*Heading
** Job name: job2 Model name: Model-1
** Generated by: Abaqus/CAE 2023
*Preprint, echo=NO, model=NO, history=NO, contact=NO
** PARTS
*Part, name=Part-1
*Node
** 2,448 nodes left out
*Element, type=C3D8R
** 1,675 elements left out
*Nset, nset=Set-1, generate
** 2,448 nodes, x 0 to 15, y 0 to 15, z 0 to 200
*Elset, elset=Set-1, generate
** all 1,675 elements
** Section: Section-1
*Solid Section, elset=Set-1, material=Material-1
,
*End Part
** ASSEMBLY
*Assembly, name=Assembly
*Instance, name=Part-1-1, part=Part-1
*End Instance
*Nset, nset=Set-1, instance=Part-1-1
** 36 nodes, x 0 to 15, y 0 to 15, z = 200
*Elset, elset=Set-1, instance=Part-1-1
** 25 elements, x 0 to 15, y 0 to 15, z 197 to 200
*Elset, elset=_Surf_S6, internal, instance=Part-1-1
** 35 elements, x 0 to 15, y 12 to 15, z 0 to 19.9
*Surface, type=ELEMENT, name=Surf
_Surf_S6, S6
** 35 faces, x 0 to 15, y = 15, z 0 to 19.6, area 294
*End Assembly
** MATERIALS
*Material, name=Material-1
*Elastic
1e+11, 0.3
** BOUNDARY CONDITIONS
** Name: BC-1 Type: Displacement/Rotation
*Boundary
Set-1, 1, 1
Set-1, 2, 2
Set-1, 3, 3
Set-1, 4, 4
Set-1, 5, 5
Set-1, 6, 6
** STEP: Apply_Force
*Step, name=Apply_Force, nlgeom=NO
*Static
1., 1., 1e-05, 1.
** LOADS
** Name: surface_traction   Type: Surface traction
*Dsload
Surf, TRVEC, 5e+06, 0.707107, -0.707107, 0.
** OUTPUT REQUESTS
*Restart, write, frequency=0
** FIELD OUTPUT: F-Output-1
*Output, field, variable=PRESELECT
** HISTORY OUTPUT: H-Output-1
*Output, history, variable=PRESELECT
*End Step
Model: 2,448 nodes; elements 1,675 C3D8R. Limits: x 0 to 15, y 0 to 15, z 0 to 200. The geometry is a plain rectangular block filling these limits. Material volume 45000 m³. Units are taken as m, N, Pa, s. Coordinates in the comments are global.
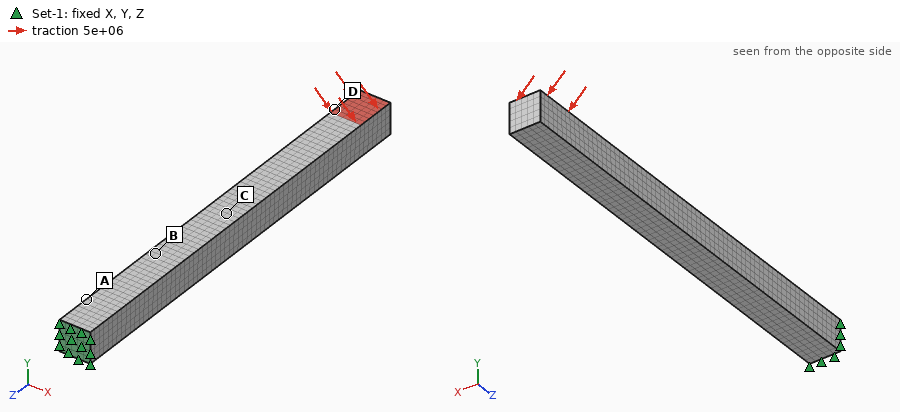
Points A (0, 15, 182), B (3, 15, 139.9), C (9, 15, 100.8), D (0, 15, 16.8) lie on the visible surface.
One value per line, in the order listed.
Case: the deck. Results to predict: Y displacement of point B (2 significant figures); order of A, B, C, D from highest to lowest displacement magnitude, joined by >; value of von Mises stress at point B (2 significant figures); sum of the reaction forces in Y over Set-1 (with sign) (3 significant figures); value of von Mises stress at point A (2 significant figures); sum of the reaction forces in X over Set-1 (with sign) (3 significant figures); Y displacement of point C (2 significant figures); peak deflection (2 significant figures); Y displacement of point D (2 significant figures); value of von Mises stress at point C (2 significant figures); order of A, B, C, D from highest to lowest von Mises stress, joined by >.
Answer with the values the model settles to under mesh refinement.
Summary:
-0.75 m
D > C > B > A
3.9e+08 Pa
1.04e+09 N
6.4e+08 Pa
-1.04e+09 N
-1.9 m
8.7 m
-5.3 m
1.4e+08 Pa
A > B > C > D
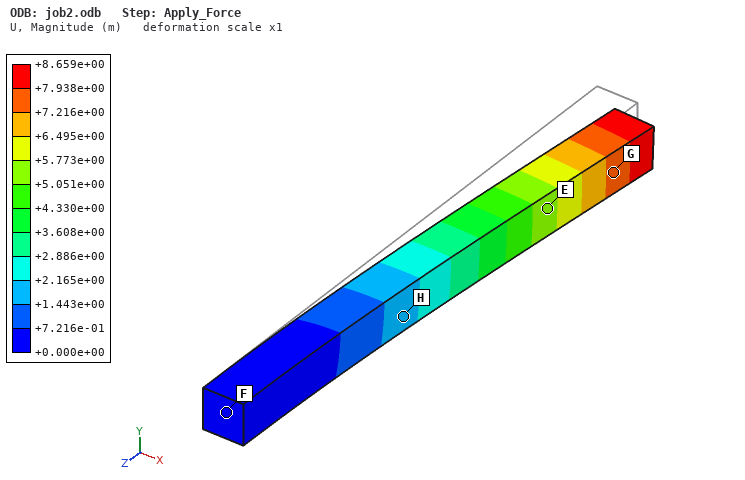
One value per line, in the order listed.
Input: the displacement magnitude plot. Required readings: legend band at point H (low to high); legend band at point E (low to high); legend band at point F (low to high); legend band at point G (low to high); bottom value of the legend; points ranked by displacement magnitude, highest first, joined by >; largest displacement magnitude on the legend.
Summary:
+1.443e+00 to +2.165e+00 m
+5.051e+00 to +5.773e+00 m
+0.000e+00 to +7.216e-01 m
+7.216e+00 to +7.938e+00 m
+0.000e+00 m
G > E > H > F
+8.659e+00 m
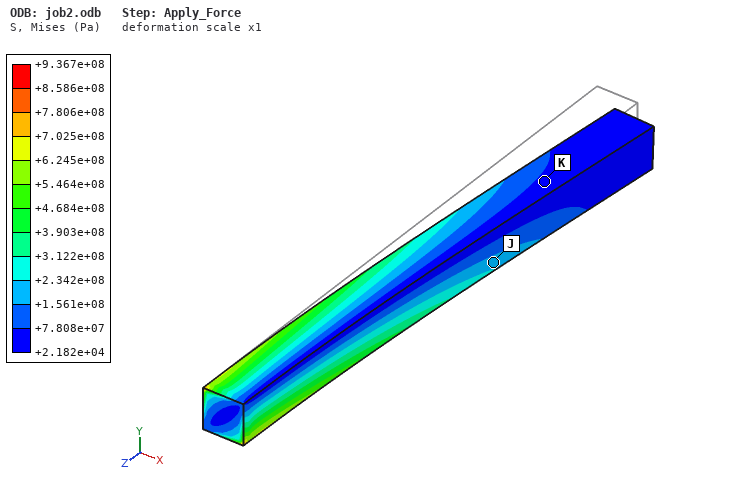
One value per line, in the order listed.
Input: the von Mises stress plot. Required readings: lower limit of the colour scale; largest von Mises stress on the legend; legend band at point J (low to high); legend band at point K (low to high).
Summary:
+2.182e+04 Pa
+9.367e+08 Pa
+1.561e+08 to +2.342e+08 Pa
+2.182e+04 to +7.808e+07 Pa
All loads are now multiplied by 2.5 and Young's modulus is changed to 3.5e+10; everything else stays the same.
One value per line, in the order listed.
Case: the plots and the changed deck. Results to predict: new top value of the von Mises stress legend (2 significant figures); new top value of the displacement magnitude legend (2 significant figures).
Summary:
2.3e+09 Pa
62 m
